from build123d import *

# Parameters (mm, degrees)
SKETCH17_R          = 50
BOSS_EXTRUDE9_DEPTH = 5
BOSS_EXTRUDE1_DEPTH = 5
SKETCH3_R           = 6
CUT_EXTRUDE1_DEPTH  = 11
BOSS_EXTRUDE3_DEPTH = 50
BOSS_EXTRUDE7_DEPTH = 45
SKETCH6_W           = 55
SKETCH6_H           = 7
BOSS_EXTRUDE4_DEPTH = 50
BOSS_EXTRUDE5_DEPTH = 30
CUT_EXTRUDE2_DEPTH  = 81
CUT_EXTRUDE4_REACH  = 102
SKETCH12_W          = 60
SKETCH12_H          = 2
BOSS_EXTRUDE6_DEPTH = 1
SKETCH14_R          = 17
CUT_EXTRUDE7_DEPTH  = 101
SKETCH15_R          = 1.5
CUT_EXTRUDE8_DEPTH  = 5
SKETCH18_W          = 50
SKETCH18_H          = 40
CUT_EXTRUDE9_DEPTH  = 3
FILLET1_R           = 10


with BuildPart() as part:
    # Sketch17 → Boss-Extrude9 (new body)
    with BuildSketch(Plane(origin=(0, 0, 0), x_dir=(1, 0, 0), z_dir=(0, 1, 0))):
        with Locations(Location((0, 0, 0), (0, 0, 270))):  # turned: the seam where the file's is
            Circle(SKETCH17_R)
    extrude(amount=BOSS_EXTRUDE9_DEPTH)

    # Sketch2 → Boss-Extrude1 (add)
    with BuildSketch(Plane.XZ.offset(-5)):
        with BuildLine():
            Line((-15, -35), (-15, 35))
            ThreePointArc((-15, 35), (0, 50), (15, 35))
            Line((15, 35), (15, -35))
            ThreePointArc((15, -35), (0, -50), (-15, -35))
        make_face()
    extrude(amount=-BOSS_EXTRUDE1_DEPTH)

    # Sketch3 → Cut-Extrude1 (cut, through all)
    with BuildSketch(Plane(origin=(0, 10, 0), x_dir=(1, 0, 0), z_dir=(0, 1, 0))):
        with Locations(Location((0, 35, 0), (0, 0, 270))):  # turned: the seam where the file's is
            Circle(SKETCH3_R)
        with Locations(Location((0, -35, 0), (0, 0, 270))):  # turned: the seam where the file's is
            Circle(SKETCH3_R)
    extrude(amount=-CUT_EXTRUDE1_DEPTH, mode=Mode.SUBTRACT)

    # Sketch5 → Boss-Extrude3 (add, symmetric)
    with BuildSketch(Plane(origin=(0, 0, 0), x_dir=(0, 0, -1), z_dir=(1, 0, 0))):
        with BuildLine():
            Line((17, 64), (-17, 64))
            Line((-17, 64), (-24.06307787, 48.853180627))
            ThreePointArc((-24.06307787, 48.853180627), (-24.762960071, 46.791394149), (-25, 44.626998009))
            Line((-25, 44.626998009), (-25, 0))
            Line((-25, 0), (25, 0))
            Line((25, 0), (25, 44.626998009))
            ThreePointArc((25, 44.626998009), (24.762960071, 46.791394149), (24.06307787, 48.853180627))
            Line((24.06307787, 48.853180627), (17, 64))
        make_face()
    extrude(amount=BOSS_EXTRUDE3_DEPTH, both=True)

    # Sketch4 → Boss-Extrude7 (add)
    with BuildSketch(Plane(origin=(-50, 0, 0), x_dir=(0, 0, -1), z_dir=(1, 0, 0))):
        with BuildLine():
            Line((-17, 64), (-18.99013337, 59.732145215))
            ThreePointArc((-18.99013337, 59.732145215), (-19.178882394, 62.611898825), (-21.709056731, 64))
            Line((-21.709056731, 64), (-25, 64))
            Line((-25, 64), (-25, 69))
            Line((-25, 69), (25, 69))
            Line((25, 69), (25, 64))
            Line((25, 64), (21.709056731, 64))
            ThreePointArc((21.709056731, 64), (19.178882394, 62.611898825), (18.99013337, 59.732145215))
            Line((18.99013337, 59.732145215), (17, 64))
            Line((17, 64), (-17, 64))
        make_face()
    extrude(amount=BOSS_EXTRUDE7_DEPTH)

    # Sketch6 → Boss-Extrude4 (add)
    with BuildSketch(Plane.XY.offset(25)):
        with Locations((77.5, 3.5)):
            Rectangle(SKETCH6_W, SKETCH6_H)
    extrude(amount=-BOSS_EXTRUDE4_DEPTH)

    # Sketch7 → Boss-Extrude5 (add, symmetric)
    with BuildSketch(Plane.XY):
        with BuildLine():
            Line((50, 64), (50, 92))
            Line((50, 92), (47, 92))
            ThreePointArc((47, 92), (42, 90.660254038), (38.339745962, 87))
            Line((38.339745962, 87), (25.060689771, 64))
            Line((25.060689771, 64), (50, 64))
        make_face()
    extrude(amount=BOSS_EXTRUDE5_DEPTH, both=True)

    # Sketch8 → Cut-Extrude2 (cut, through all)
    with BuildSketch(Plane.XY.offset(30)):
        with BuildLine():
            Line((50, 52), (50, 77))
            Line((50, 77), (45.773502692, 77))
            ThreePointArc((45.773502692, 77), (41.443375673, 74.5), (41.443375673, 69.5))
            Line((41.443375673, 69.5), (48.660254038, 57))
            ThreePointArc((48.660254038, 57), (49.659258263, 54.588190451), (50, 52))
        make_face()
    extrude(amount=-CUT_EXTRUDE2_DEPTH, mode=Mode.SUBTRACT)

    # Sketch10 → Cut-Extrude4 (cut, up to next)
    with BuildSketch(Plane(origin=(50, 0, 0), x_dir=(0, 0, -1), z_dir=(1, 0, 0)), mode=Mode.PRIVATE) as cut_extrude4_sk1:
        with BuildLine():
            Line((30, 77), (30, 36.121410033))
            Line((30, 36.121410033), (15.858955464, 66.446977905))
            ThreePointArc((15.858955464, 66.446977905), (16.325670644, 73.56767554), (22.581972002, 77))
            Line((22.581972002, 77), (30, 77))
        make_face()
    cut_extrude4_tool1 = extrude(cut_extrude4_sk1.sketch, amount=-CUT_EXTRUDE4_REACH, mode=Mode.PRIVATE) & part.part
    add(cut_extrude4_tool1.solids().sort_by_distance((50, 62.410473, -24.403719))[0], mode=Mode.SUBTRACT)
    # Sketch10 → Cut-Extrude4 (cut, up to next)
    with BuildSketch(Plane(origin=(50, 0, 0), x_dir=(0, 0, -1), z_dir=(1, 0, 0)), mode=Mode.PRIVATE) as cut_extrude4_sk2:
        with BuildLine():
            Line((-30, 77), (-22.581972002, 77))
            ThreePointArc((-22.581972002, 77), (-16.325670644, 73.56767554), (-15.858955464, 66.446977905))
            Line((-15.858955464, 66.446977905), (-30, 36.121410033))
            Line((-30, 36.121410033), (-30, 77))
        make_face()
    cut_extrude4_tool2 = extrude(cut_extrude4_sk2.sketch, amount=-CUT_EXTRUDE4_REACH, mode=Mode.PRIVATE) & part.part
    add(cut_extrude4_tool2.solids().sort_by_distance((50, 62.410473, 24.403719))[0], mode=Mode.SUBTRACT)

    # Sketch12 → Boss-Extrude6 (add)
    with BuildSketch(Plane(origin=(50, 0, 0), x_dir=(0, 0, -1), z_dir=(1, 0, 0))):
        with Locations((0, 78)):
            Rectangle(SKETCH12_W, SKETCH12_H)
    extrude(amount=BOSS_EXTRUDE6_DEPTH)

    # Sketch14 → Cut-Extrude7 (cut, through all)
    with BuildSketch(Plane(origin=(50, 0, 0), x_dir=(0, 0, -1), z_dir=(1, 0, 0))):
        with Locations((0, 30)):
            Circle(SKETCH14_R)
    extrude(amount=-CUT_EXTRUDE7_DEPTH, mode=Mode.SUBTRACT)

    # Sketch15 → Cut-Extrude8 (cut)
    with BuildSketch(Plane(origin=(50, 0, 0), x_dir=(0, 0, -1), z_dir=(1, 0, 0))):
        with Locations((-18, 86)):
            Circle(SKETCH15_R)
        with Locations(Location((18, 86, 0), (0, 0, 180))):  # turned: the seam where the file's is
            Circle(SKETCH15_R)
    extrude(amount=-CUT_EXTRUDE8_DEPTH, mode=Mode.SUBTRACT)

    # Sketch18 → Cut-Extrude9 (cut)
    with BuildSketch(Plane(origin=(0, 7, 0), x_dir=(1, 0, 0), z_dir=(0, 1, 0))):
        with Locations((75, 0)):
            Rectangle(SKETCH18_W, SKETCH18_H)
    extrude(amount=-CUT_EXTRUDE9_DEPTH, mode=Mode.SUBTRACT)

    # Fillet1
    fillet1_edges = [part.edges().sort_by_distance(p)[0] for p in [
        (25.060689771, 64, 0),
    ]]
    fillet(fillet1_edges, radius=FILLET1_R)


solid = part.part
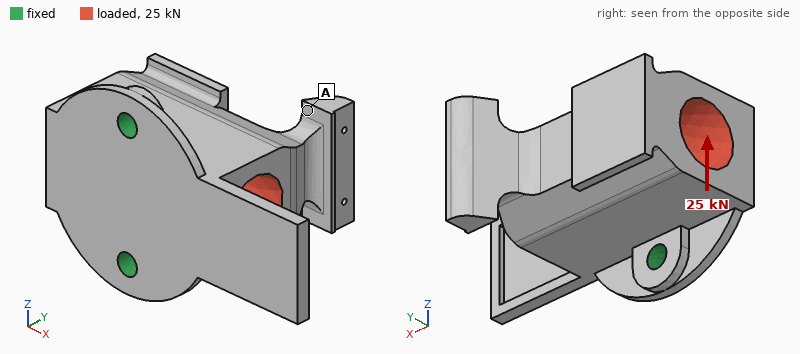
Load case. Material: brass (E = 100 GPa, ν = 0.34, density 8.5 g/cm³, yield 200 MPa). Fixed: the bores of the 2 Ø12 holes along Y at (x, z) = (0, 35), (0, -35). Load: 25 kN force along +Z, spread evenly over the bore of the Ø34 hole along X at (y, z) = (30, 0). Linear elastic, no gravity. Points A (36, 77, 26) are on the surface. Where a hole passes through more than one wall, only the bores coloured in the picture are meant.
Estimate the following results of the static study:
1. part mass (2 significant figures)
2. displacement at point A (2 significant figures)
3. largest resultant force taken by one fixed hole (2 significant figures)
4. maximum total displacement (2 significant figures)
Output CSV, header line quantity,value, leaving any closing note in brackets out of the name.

quantity,value
part mass,2.3 kg
displacement at point A,85 µm
largest resultant force taken by one fixed hole,17 kN
maximum total displacement,96 µm
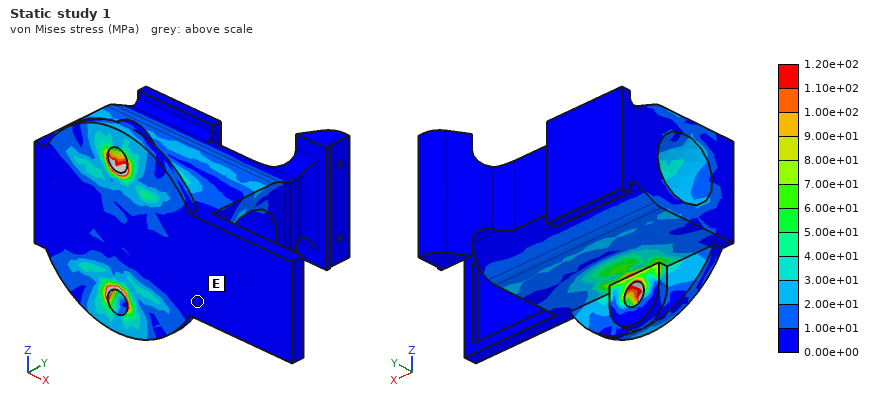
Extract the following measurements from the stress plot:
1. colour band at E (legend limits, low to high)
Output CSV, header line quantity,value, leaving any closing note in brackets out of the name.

quantity,value
colour band at E,0.00e+00 to 1.00e+01 MPa
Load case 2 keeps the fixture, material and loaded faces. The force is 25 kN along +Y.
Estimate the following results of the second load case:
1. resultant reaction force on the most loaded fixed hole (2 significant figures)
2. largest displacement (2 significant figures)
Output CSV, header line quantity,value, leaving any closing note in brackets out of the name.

quantity,value
resultant reaction force on the most loaded fixed hole,13 kN
largest displacement,44 µm
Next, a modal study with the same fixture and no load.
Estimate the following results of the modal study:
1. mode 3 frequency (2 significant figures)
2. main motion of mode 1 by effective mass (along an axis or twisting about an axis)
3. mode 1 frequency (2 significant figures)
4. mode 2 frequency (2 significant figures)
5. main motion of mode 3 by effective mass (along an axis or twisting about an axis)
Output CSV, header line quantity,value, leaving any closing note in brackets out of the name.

quantity,value
mode 3 frequency,1800 Hz
main motion of mode 1 by effective mass,along X
mode 1 frequency,630 Hz
mode 2 frequency,950 Hz
main motion of mode 3 by effective mass,along Z
